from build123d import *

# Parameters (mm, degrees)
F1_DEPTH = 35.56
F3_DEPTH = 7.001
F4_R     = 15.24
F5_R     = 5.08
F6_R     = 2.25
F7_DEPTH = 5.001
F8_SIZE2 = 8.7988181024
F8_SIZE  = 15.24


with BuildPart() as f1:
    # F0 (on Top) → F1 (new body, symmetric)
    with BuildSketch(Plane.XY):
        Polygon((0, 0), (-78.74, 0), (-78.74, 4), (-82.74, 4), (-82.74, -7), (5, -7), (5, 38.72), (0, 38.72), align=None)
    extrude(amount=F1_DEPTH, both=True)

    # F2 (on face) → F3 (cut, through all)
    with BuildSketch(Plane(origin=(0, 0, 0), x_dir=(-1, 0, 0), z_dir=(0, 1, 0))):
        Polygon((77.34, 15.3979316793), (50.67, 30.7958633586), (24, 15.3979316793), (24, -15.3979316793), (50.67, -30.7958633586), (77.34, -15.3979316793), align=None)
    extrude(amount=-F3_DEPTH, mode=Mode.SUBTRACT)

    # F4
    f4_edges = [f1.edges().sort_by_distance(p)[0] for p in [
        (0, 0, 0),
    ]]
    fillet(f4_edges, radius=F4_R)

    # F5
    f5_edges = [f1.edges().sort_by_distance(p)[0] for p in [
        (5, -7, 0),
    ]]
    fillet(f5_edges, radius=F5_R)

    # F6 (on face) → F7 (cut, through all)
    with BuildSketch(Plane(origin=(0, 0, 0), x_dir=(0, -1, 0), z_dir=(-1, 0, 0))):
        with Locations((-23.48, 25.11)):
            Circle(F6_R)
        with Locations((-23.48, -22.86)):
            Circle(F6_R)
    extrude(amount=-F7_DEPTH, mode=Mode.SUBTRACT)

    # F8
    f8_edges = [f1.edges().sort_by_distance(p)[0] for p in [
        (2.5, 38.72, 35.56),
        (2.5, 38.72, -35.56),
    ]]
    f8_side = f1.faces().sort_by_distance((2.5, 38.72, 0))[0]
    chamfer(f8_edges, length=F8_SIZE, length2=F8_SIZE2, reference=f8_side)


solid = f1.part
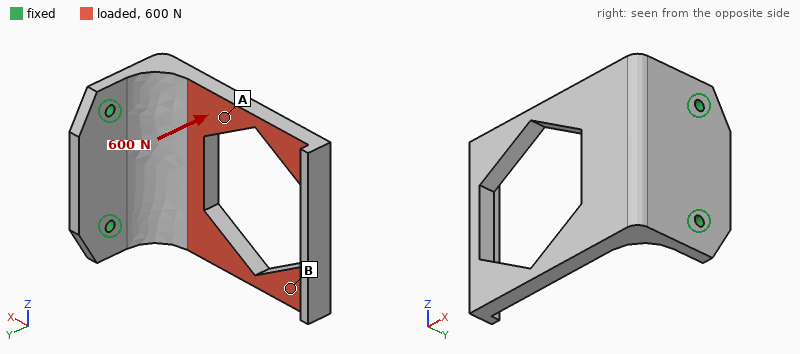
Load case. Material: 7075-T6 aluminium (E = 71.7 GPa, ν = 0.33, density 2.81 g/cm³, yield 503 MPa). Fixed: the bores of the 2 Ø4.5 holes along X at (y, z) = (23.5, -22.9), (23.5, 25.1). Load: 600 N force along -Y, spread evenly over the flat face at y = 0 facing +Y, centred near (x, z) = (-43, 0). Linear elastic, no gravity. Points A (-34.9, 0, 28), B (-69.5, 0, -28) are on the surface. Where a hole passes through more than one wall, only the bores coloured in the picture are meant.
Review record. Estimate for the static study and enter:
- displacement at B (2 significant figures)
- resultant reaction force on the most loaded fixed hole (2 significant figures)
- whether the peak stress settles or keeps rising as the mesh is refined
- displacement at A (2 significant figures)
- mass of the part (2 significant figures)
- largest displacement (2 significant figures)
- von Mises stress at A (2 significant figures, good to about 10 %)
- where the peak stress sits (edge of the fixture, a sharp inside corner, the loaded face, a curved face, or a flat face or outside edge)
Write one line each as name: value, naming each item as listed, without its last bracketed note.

displacement at B: 0.95 mm
resultant reaction force on the most loaded fixed hole: 320 N
whether the peak stress settles or keeps rising as the mesh is refined: keeps rising
displacement at A: 0.41 mm
mass of the part: 120 g
largest displacement: 1.2 mm
von Mises stress at A: 39 MPa
where the peak stress sits: edge of the fixture
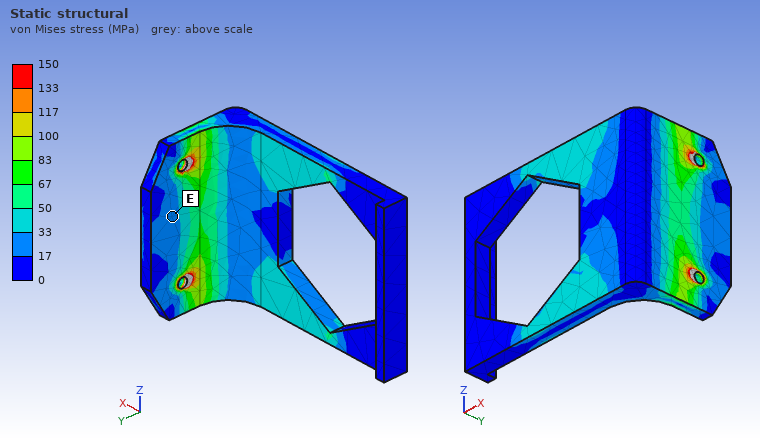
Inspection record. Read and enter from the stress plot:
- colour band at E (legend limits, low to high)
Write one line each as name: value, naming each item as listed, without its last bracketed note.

colour band at E: 17 to 33 MPa
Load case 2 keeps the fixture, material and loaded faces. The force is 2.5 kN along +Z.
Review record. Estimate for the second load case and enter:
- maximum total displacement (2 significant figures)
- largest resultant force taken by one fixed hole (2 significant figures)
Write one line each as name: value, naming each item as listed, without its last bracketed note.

maximum total displacement: 0.75 mm
largest resultant force taken by one fixed hole: 2.8 kN
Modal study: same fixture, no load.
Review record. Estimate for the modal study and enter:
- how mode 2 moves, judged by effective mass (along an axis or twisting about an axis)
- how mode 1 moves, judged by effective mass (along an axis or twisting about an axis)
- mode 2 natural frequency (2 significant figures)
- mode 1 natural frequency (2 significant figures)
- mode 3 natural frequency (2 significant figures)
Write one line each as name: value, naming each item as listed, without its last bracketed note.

how mode 2 moves, judged by effective mass: along Z
how mode 1 moves, judged by effective mass: along Y
mode 2 natural frequency: 1300 Hz
mode 1 natural frequency: 510 Hz
mode 3 natural frequency: 1800 Hz
